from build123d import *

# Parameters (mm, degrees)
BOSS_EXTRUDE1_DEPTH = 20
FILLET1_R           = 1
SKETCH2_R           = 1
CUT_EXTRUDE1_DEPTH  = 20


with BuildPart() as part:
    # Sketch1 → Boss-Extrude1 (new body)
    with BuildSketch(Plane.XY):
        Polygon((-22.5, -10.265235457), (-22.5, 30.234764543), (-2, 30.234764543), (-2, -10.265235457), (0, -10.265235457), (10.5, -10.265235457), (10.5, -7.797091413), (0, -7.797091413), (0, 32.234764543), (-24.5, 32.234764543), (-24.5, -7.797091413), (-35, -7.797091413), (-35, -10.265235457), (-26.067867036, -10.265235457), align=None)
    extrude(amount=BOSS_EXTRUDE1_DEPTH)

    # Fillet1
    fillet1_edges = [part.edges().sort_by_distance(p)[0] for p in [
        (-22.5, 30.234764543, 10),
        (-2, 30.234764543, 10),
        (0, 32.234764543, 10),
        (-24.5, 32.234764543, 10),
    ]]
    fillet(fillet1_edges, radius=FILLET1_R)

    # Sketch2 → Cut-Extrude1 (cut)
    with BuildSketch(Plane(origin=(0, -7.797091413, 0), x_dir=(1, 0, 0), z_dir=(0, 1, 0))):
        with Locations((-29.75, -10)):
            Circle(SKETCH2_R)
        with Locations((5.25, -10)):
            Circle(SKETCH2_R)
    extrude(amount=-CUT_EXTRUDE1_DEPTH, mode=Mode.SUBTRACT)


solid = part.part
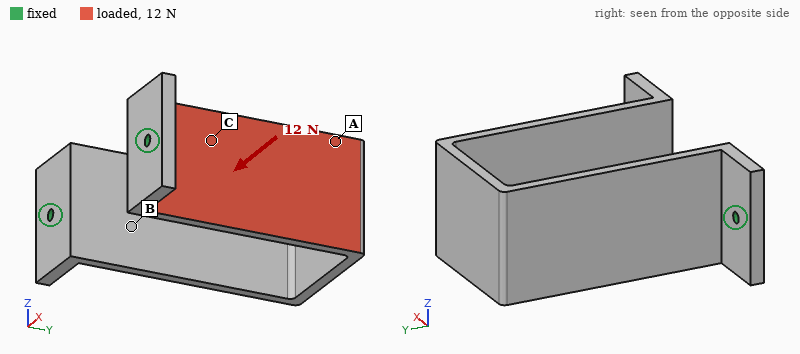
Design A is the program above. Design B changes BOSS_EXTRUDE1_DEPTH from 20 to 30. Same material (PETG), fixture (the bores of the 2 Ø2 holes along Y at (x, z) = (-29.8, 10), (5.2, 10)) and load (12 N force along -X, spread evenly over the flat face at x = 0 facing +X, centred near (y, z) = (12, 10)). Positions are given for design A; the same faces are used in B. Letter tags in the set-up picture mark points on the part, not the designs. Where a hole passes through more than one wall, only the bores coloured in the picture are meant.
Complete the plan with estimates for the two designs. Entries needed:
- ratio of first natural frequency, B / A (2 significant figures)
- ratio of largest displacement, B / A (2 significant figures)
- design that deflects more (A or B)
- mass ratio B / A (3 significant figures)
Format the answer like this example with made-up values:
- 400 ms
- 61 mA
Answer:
- 0.95
- 0.73
- A
- 1.50
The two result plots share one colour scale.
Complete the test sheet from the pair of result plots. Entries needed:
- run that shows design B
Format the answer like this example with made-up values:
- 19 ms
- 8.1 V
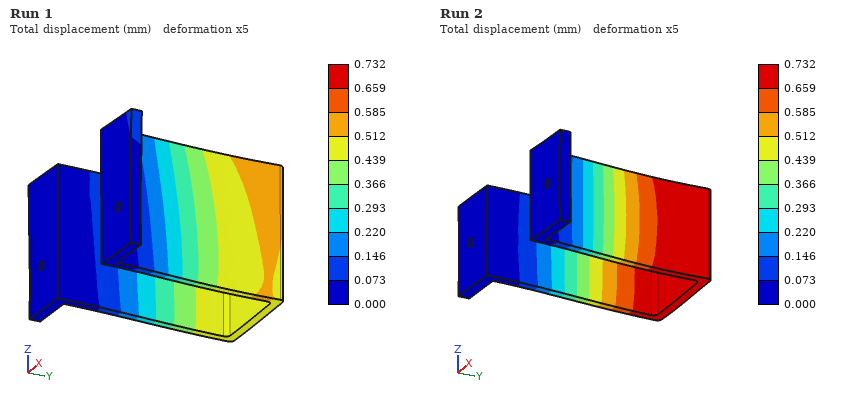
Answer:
- Run 1
